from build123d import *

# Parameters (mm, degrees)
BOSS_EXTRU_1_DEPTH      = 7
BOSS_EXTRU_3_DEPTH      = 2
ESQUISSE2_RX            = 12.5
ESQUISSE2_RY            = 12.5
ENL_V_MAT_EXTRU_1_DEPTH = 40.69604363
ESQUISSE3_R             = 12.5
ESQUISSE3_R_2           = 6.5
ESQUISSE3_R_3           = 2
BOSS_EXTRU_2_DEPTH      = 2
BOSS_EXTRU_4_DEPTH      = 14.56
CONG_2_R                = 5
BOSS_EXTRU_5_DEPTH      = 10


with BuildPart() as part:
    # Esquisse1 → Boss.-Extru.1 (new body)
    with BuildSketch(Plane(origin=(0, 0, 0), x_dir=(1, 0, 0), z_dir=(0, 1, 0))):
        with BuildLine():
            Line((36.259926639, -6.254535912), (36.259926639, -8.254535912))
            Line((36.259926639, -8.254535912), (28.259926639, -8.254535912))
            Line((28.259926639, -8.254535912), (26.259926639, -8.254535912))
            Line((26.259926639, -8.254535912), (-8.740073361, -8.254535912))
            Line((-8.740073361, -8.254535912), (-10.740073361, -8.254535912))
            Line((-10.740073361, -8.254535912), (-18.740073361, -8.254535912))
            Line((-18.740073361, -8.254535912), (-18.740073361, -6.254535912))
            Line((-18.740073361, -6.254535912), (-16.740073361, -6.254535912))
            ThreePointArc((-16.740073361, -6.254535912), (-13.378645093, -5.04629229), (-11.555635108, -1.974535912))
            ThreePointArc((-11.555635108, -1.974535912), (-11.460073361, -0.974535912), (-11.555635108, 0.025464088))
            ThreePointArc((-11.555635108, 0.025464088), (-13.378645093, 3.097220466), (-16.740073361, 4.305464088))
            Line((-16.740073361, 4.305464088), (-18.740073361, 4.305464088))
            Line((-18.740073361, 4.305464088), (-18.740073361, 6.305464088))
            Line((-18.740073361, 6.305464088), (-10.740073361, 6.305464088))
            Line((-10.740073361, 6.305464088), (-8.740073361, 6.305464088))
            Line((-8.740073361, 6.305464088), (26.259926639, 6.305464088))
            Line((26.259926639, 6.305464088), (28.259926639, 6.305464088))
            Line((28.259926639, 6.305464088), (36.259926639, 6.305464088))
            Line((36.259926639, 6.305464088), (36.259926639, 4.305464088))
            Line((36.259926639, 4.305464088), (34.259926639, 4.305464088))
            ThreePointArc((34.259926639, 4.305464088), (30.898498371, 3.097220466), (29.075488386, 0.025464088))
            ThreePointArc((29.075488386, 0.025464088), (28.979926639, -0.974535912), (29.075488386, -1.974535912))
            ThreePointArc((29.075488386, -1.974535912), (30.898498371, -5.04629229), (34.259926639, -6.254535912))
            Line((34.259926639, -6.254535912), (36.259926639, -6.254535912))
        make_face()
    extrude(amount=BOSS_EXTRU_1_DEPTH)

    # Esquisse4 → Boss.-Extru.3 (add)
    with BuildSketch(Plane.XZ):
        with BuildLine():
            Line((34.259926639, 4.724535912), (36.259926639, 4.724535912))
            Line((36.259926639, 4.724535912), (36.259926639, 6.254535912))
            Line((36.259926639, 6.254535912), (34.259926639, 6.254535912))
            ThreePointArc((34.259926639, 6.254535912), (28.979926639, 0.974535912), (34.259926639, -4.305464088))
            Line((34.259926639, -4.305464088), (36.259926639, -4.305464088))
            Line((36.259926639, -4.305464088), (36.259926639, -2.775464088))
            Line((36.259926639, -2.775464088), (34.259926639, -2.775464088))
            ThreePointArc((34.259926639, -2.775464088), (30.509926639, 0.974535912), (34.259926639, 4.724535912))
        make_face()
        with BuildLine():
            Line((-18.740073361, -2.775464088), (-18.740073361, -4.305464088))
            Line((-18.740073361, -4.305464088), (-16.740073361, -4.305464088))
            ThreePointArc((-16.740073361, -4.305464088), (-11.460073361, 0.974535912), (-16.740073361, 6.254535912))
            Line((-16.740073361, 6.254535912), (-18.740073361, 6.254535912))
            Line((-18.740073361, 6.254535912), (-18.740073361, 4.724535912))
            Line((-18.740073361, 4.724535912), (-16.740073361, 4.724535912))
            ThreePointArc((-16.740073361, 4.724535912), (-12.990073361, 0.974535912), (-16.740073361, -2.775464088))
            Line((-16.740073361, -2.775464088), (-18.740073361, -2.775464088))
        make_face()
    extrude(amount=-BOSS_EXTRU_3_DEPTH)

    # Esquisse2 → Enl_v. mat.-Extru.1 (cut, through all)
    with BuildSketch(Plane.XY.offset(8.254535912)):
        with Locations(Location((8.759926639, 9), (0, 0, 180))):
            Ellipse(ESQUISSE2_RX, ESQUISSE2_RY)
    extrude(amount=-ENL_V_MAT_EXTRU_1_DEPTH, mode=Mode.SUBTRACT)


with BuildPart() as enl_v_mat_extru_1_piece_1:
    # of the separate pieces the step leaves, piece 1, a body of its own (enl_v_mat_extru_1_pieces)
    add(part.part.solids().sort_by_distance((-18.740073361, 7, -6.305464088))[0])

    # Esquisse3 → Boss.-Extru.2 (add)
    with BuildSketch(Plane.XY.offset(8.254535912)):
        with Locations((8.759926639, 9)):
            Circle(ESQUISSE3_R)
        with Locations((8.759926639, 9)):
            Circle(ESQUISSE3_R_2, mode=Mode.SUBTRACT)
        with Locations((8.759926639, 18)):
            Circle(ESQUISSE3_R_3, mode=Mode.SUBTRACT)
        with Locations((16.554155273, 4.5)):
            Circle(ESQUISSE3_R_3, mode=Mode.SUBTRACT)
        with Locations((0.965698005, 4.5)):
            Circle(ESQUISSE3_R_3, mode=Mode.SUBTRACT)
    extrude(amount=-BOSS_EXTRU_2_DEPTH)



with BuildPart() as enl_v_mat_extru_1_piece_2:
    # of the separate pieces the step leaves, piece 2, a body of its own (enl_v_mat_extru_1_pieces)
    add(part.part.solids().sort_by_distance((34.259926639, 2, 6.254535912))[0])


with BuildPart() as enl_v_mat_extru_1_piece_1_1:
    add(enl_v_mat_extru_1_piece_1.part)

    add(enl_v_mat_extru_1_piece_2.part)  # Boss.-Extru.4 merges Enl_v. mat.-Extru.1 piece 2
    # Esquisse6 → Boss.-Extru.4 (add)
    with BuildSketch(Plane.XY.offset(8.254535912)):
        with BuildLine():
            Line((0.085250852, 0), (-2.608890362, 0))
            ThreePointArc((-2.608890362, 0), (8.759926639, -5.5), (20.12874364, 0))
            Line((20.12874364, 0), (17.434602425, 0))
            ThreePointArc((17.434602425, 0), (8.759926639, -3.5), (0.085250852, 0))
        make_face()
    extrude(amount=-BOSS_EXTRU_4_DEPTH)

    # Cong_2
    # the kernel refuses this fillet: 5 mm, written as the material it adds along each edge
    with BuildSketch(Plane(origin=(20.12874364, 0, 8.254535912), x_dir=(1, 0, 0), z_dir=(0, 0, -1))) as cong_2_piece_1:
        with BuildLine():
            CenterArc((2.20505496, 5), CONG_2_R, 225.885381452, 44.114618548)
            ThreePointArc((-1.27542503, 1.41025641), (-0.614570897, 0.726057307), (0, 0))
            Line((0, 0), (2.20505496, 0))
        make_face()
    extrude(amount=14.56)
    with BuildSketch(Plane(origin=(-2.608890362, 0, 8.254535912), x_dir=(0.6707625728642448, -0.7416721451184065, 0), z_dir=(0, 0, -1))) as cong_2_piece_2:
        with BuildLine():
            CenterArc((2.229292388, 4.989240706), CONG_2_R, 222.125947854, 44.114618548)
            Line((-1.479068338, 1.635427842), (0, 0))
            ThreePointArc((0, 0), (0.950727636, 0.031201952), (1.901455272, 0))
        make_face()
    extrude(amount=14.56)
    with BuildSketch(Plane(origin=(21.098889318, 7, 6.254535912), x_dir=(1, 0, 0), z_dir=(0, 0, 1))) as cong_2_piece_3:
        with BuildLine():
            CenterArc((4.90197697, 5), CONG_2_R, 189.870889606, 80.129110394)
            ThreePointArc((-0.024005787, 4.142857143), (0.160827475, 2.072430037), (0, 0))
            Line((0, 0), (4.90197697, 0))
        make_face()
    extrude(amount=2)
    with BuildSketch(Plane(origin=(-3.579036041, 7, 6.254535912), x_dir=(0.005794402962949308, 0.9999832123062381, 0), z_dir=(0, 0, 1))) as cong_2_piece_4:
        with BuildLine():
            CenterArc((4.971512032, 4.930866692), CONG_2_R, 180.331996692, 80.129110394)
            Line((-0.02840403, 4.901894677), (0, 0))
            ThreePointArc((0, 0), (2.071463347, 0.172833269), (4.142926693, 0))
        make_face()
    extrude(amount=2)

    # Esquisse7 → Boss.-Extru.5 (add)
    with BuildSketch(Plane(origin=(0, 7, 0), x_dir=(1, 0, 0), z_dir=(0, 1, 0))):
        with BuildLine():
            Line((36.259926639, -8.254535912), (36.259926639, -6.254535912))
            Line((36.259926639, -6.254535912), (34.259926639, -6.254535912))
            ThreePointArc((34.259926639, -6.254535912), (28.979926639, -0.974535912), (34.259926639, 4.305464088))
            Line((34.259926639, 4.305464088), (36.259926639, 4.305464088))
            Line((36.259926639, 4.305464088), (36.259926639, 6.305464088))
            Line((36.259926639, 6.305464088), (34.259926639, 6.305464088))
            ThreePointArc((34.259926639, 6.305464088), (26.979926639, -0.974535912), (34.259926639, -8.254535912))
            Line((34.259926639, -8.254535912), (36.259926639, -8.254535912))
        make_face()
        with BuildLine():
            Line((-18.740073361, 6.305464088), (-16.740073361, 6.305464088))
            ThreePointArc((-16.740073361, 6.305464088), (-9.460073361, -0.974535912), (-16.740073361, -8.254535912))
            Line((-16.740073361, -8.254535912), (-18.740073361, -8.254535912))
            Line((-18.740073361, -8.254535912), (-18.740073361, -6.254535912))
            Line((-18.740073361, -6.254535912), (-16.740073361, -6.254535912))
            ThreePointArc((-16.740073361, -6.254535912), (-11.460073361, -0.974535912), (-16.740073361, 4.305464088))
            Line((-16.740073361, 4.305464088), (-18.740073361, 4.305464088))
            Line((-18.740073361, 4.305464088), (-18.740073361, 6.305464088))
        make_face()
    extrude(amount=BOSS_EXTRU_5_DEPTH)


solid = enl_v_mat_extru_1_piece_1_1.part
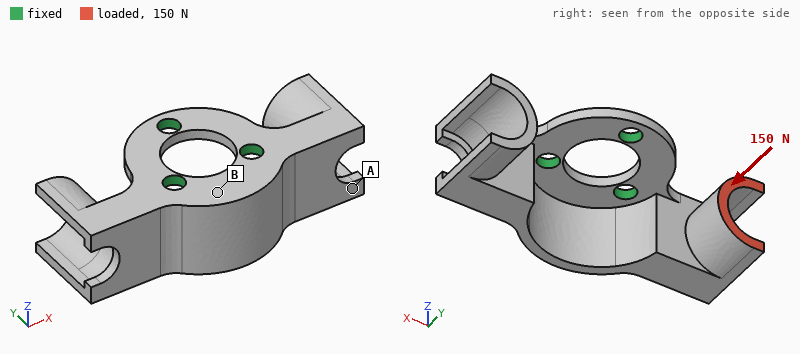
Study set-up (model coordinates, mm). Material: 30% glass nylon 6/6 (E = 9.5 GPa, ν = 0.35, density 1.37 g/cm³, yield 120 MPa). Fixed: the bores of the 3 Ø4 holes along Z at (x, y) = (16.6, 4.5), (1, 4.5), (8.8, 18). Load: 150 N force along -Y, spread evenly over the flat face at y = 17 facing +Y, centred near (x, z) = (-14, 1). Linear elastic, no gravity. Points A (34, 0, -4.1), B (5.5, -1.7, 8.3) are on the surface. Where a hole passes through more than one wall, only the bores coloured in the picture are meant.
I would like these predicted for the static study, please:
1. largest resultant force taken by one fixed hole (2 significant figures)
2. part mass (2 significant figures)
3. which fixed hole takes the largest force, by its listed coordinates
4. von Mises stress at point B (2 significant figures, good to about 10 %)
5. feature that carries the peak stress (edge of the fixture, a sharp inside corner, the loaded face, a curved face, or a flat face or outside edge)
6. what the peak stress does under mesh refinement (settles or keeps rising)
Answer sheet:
140 N
6.6 g
(1, 4.5)
14 MPa
edge of the fixture
keeps rising
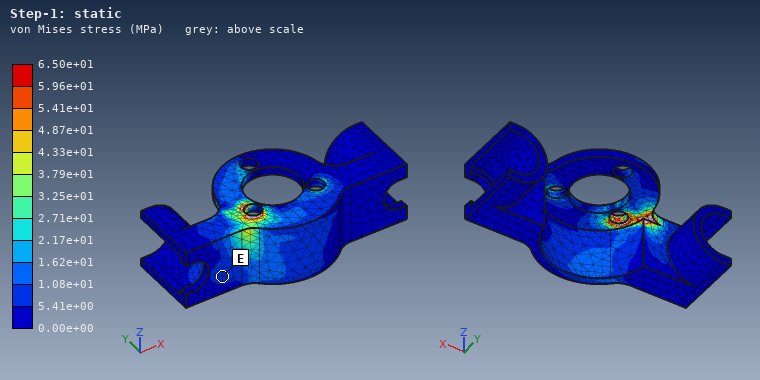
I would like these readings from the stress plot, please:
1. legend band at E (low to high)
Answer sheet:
5.41e+00 to 1.08e+01 MPa
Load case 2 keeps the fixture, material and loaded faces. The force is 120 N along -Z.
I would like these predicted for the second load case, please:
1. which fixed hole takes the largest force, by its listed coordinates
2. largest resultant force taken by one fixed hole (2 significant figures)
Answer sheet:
(1, 4.5)
190 N
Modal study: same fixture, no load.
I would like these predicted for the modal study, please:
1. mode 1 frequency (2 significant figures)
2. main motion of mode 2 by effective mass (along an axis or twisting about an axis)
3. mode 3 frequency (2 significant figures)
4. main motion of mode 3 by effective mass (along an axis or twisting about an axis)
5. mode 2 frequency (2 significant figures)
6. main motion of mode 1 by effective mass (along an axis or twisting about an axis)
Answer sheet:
2000 Hz
along Y
2700 Hz
along Z
2400 Hz
along X
